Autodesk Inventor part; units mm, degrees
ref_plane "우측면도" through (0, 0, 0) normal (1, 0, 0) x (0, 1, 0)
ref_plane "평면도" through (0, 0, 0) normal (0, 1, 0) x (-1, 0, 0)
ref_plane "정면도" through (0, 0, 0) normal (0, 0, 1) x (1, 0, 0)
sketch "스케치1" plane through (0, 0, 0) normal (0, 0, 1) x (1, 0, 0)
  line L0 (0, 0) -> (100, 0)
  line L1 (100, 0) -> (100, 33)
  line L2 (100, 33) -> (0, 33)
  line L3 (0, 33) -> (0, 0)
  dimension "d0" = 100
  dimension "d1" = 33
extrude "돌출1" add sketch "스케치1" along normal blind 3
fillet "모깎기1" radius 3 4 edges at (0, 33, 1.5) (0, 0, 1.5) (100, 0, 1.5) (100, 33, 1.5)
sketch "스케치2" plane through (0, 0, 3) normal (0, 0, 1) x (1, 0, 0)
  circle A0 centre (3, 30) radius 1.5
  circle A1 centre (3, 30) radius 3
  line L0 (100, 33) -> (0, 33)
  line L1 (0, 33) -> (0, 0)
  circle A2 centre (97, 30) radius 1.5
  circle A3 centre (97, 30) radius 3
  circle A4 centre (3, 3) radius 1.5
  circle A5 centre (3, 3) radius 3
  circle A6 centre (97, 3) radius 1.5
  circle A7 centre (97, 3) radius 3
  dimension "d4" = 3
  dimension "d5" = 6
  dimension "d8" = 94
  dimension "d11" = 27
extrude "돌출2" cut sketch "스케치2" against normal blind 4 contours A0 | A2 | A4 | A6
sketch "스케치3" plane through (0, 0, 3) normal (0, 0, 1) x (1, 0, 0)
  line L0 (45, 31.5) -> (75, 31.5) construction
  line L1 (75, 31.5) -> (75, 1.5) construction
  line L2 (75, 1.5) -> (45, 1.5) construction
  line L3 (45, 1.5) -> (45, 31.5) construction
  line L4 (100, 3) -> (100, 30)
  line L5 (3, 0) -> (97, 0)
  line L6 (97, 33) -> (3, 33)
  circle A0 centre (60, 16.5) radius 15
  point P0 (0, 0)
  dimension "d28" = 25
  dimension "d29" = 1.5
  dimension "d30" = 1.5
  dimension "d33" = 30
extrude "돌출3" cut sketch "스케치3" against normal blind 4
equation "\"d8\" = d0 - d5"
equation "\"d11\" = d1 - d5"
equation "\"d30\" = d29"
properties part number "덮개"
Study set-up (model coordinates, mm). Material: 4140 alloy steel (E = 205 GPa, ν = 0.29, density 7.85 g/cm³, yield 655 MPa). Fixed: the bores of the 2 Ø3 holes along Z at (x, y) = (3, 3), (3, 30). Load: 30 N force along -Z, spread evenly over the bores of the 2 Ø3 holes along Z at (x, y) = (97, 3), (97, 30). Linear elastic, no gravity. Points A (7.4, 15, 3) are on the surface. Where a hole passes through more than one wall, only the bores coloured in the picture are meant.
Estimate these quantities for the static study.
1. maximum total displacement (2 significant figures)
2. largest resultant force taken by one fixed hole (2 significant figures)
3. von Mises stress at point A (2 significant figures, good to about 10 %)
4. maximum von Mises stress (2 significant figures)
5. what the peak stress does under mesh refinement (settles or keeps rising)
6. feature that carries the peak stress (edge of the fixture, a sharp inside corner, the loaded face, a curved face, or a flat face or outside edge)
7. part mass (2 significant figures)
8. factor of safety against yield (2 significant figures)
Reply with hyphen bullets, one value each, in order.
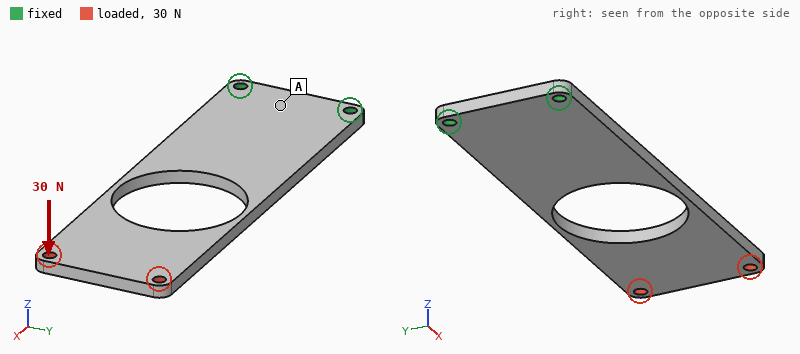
- 1.1 mm
- 15 N
- 34 MPa
- 270 MPa
- settles
- a curved face
- 60 g
- 2.5
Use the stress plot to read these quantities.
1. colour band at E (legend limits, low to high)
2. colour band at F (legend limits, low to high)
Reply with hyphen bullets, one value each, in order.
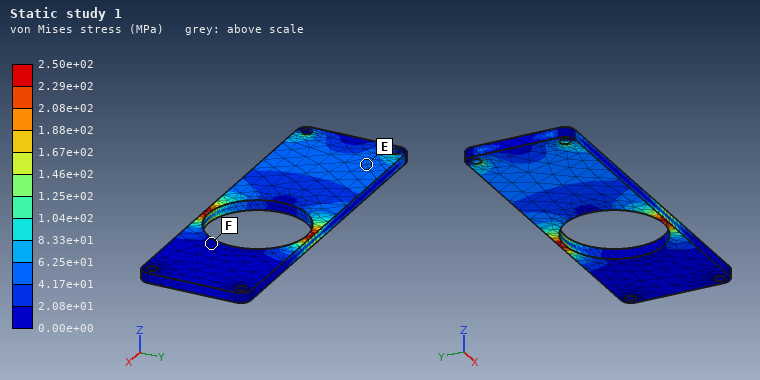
- 4.17e+01 to 6.25e+01 MPa
- 0.00e+00 to 2.08e+01 MPa
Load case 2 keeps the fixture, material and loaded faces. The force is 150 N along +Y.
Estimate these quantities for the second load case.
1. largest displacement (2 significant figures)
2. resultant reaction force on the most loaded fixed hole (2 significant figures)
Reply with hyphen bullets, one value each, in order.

- 89 µm
- 520 N
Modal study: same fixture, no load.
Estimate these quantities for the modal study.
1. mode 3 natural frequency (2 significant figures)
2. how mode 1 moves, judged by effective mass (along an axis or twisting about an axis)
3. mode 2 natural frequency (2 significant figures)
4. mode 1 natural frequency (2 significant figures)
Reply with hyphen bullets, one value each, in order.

- 1300 Hz
- along Z
- 1300 Hz
- 230 Hz
